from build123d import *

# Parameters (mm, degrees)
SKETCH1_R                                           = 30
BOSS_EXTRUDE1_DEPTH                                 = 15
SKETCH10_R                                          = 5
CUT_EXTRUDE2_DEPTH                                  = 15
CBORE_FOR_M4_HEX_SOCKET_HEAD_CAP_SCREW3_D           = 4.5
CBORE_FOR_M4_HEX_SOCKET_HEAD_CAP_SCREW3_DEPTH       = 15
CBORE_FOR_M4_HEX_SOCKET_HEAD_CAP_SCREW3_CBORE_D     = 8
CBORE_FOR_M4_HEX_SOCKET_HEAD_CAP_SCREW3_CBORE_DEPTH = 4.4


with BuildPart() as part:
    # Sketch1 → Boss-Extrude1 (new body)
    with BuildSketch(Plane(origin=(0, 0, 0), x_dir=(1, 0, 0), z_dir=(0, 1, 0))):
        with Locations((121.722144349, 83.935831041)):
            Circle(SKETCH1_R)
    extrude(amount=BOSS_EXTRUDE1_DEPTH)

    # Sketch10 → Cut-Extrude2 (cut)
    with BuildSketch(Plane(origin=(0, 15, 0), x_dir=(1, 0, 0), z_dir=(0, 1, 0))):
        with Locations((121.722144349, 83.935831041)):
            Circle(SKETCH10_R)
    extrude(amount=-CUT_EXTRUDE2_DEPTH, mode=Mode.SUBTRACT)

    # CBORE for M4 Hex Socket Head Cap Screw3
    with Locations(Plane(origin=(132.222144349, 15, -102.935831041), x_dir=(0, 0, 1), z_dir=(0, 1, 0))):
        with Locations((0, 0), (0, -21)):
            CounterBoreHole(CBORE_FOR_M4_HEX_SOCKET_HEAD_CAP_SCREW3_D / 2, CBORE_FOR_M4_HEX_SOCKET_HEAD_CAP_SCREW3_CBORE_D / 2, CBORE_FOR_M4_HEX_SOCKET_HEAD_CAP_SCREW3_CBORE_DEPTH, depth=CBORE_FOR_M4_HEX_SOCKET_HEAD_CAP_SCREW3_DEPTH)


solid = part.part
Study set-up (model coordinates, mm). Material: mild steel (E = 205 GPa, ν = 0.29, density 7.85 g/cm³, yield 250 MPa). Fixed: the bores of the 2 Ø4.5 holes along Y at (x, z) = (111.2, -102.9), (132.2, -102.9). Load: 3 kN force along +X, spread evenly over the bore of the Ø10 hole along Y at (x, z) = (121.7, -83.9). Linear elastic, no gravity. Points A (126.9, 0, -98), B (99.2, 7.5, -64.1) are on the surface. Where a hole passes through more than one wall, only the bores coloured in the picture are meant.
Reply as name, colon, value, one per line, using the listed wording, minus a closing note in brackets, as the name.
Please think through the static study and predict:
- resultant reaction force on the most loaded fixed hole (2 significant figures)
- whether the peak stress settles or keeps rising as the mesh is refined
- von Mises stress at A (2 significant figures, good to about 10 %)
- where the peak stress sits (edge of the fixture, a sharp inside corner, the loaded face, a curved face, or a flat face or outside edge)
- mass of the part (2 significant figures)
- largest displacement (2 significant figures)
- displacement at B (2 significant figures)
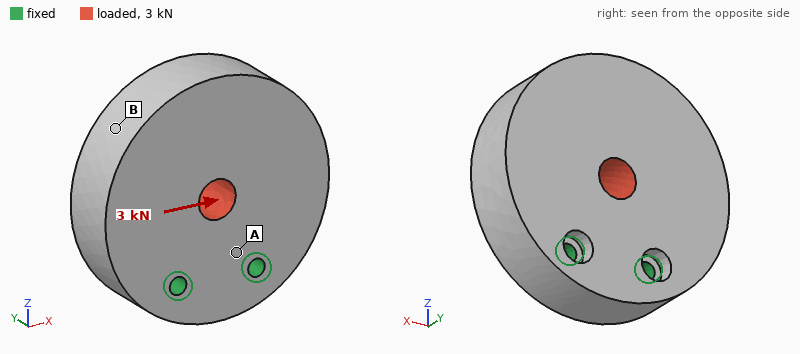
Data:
resultant reaction force on the most loaded fixed hole: 2.8 kN
whether the peak stress settles or keeps rising as the mesh is refined: keeps rising
von Mises stress at A: 17 MPa
where the peak stress sits: edge of the fixture
mass of the part: 320 g
largest displacement: 5.1 µm
displacement at B: 4.7 µm
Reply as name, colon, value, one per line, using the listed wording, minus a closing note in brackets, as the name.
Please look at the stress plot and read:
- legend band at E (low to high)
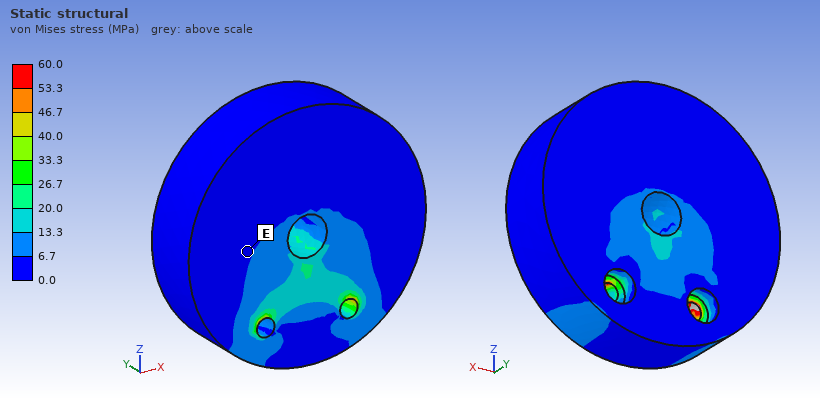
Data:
legend band at E: 0.0 to 6.7 MPa
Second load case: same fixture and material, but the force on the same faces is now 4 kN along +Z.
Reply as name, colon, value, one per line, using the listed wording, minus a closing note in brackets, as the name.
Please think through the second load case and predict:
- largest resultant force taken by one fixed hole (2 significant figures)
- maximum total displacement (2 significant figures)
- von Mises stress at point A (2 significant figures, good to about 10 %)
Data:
largest resultant force taken by one fixed hole: 2.0 kN
maximum total displacement: 2.8 µm
von Mises stress at point A: 5.9 MPa
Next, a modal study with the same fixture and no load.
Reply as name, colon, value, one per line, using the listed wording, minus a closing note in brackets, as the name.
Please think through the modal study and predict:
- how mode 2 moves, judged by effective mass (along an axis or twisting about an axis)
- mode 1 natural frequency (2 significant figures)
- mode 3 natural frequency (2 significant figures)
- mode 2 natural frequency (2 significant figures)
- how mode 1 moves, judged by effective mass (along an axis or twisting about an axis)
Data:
how mode 2 moves, judged by effective mass: along X
mode 1 natural frequency: 3800 Hz
mode 3 natural frequency: 8600 Hz
mode 2 natural frequency: 7300 Hz
how mode 1 moves, judged by effective mass: along Y
